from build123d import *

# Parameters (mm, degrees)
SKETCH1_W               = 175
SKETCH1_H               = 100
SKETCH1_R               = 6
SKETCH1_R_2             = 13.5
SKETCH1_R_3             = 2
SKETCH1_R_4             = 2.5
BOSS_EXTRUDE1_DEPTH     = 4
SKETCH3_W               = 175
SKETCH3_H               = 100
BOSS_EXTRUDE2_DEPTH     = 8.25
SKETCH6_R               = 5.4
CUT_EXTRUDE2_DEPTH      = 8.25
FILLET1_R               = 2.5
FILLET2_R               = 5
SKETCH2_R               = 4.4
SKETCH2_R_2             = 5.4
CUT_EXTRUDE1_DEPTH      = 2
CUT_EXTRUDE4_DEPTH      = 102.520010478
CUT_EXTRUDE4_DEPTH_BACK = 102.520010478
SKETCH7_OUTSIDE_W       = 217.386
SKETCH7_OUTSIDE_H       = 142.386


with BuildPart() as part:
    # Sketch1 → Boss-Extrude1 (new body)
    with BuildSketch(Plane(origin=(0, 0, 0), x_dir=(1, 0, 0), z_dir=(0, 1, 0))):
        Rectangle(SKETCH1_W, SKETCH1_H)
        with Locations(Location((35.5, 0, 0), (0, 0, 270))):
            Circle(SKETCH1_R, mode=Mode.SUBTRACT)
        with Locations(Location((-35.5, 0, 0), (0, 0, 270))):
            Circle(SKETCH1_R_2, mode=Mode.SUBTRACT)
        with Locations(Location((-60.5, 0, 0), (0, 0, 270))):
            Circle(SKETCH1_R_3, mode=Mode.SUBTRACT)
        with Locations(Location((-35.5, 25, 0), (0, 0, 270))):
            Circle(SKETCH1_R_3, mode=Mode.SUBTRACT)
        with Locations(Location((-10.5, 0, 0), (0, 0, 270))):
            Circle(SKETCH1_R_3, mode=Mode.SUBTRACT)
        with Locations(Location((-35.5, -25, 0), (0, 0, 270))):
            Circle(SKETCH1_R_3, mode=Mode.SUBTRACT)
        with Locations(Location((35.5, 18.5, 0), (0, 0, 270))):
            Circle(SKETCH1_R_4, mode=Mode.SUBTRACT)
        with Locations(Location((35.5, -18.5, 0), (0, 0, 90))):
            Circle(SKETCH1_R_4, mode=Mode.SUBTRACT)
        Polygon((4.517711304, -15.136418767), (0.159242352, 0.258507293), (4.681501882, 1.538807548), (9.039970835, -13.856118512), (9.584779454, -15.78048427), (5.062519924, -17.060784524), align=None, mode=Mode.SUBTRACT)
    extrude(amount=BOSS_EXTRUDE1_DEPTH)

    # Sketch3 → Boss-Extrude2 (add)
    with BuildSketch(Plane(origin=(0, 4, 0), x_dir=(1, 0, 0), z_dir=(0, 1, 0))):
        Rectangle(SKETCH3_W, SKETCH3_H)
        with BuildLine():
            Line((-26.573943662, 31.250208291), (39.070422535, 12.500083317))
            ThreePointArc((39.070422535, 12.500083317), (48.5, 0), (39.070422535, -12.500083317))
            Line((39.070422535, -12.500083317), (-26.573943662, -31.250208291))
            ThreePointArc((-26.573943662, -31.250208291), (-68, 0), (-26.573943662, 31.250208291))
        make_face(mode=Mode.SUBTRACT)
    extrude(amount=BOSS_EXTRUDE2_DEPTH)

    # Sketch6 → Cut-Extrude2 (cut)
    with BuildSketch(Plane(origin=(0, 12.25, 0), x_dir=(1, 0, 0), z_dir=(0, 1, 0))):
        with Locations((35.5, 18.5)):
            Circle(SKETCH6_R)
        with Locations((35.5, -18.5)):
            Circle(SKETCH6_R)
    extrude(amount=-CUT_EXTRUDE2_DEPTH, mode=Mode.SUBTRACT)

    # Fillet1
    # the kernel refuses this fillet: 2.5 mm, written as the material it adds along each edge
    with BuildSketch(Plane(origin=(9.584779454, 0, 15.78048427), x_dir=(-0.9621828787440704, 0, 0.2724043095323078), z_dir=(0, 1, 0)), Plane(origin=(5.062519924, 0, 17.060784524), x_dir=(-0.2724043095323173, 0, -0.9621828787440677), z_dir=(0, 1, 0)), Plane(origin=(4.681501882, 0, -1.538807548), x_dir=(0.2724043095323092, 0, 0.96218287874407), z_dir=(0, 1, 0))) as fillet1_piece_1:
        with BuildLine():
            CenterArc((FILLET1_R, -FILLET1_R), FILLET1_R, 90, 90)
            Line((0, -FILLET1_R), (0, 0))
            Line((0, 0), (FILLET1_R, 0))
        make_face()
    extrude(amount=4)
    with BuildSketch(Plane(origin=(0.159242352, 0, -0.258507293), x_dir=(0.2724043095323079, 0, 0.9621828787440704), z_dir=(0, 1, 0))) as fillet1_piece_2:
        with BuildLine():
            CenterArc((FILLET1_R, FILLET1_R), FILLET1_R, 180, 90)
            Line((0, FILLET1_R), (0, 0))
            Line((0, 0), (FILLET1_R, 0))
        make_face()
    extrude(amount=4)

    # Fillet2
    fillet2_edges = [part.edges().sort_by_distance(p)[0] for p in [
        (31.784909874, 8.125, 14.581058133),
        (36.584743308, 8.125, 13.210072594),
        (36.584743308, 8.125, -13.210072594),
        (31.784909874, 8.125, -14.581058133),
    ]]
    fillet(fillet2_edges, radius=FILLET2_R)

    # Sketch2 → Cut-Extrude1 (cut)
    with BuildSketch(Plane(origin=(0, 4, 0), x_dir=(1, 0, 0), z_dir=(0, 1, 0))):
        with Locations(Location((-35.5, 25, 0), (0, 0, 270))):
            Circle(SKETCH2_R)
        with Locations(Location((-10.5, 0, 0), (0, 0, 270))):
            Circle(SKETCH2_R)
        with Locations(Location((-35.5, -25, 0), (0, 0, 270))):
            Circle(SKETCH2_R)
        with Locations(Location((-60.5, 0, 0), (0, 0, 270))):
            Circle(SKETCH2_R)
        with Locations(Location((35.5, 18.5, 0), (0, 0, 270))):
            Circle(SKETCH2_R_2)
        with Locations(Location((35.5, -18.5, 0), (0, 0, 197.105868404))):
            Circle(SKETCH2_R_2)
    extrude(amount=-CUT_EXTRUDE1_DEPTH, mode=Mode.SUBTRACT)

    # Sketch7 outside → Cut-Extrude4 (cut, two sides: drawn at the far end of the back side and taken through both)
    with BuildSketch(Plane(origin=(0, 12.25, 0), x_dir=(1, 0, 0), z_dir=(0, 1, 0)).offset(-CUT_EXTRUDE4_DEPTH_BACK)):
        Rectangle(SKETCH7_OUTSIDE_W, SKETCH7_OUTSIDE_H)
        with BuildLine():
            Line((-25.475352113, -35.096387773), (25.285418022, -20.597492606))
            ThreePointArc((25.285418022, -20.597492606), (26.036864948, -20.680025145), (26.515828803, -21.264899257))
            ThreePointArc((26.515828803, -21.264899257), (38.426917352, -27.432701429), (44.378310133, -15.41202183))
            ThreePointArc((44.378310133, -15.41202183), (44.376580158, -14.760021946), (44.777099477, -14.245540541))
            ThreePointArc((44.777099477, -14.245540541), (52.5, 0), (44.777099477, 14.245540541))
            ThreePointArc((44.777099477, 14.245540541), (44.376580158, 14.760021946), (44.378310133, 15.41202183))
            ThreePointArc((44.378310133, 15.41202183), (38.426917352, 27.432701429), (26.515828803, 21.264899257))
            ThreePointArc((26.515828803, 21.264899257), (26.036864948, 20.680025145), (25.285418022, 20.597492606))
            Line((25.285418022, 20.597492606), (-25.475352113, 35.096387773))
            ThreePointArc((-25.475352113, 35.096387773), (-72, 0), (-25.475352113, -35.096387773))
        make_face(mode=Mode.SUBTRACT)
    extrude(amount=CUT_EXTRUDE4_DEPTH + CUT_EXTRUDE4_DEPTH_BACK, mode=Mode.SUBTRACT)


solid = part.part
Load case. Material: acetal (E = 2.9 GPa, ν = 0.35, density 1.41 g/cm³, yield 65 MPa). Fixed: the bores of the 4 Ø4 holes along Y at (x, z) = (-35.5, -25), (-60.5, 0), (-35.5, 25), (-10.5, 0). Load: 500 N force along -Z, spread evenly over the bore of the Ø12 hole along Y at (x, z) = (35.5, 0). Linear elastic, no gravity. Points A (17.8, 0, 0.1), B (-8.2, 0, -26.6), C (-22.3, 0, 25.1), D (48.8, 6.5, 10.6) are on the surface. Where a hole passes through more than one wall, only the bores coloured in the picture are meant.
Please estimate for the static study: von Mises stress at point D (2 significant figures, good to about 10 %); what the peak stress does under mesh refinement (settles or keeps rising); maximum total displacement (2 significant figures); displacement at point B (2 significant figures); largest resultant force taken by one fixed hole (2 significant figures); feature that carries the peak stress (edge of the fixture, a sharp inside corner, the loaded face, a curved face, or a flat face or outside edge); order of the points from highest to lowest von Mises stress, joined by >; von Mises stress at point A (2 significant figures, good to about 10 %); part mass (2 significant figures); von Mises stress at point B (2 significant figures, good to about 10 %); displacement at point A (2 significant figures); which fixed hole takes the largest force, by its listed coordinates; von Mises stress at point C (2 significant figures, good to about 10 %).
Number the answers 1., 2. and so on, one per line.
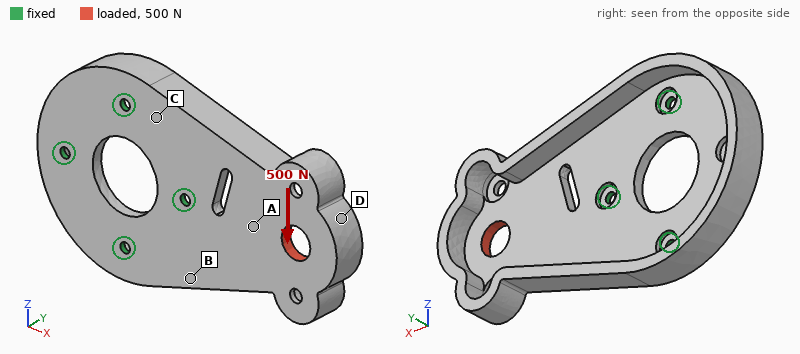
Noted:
1. 1.7 MPa
2. keeps rising
3. 0.50 mm
4. 0.12 mm
5. 510 N
6. edge of the fixture
7. B > C > A > D
8. 3.8 MPa
9. 48 g
10. 8.2 MPa
11. 0.21 mm
12. (-10.5, 0)
13. 6.1 MPa
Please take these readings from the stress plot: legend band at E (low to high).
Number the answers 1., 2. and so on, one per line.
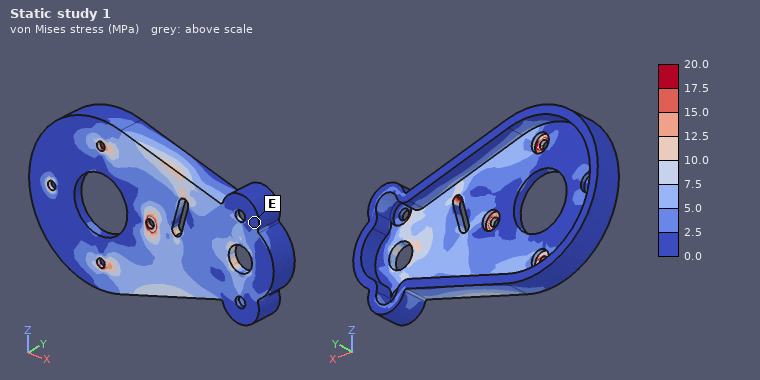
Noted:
1. 0.0 to 2.5 MPa
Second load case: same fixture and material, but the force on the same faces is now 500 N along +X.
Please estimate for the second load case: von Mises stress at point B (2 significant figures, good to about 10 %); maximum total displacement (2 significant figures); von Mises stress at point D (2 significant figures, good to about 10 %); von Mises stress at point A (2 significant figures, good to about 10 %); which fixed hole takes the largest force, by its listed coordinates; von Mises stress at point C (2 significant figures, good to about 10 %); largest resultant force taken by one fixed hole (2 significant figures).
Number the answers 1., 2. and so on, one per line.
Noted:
1. 2.0 MPa
2. 0.17 mm
3. 0.96 MPa
4. 3.7 MPa
5. (-10.5, 0)
6. 1.9 MPa
7. 220 N
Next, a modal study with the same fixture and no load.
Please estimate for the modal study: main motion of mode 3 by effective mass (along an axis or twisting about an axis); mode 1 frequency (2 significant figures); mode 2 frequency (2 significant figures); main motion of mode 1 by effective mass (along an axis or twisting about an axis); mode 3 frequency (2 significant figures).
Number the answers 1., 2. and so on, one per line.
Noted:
1. along Z
2. 300 Hz
3. 510 Hz
4. along Y
5. 1400 Hz
